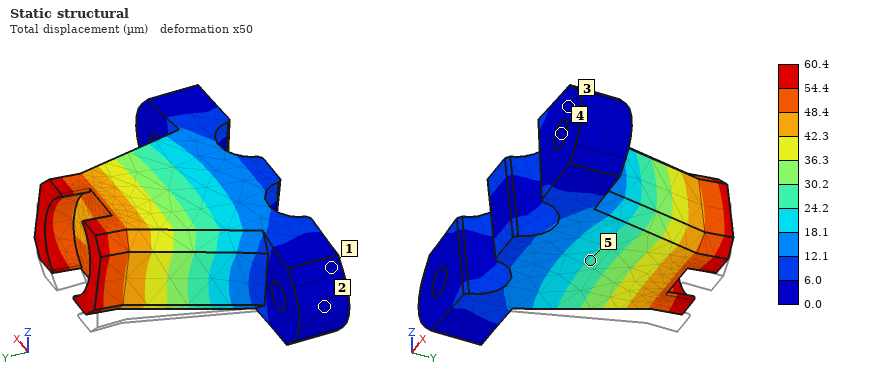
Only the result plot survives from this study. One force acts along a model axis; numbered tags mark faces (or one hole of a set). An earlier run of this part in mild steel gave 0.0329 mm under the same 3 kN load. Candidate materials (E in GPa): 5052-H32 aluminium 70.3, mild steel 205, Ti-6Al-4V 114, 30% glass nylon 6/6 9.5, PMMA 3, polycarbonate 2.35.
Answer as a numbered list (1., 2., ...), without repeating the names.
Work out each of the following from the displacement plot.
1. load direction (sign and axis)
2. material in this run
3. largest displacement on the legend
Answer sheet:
1. +Z
2. Ti-6Al-4V
3. 60.4 µm
